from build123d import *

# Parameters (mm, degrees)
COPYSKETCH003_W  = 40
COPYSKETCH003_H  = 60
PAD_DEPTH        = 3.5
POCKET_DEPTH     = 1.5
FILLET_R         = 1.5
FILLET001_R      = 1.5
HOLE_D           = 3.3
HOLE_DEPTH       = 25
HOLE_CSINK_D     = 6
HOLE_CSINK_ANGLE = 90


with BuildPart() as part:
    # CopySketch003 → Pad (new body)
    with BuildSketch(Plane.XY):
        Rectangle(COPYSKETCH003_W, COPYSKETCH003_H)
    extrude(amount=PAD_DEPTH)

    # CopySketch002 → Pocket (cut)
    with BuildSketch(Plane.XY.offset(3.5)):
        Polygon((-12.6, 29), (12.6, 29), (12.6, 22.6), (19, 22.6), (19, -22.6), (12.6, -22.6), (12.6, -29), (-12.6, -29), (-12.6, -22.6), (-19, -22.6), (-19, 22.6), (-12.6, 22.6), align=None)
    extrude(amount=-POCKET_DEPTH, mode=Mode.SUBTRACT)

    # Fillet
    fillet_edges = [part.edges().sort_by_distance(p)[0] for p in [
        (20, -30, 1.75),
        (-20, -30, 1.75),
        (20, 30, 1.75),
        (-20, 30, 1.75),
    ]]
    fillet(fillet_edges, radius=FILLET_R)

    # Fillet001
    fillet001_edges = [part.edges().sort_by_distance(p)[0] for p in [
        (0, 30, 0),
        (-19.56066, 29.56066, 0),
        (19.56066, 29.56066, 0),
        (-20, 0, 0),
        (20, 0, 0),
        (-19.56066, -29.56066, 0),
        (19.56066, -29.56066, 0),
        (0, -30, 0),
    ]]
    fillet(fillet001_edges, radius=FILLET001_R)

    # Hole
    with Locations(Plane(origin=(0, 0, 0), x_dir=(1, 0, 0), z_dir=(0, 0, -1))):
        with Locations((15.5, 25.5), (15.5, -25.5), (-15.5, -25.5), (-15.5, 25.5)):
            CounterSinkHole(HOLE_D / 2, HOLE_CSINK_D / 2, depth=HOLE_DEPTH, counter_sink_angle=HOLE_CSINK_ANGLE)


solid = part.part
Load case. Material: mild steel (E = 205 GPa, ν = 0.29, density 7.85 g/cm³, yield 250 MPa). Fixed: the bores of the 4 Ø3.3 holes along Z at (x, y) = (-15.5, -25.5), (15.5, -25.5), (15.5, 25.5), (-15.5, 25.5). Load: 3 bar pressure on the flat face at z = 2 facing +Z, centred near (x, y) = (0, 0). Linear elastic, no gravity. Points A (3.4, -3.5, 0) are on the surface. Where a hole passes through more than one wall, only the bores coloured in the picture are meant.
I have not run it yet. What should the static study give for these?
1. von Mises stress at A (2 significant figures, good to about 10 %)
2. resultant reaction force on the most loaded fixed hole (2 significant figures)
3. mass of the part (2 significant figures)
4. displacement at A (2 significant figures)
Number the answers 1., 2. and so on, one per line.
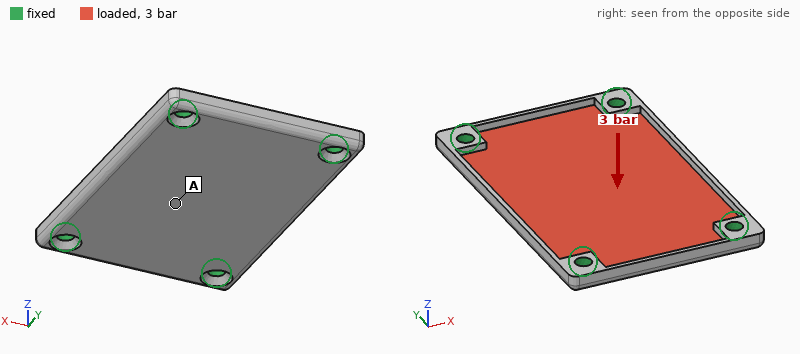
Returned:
1. 40 MPa
2. 240 N
3. 40 g
4. 37 µm
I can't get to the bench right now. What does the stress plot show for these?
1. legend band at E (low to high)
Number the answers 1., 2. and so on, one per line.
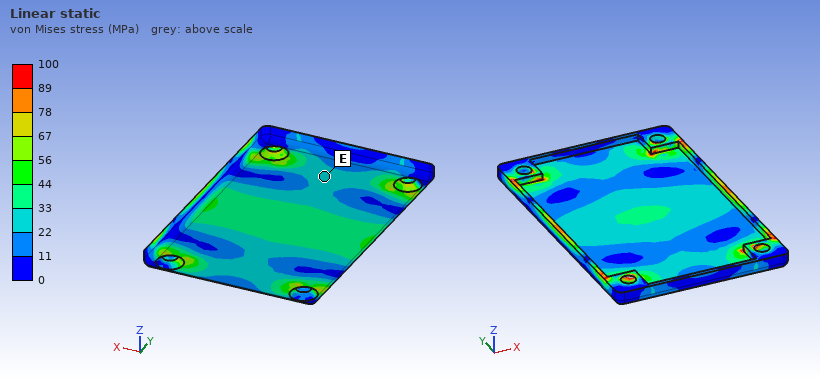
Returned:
1. 22 to 33 MPa
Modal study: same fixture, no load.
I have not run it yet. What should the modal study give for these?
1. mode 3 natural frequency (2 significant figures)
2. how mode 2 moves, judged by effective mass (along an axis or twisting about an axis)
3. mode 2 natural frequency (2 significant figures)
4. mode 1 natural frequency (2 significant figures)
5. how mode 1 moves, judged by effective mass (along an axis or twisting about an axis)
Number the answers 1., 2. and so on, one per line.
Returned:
1. 9700 Hz
2. twisting about Y
3. 6100 Hz
4. 4100 Hz
5. along Z
